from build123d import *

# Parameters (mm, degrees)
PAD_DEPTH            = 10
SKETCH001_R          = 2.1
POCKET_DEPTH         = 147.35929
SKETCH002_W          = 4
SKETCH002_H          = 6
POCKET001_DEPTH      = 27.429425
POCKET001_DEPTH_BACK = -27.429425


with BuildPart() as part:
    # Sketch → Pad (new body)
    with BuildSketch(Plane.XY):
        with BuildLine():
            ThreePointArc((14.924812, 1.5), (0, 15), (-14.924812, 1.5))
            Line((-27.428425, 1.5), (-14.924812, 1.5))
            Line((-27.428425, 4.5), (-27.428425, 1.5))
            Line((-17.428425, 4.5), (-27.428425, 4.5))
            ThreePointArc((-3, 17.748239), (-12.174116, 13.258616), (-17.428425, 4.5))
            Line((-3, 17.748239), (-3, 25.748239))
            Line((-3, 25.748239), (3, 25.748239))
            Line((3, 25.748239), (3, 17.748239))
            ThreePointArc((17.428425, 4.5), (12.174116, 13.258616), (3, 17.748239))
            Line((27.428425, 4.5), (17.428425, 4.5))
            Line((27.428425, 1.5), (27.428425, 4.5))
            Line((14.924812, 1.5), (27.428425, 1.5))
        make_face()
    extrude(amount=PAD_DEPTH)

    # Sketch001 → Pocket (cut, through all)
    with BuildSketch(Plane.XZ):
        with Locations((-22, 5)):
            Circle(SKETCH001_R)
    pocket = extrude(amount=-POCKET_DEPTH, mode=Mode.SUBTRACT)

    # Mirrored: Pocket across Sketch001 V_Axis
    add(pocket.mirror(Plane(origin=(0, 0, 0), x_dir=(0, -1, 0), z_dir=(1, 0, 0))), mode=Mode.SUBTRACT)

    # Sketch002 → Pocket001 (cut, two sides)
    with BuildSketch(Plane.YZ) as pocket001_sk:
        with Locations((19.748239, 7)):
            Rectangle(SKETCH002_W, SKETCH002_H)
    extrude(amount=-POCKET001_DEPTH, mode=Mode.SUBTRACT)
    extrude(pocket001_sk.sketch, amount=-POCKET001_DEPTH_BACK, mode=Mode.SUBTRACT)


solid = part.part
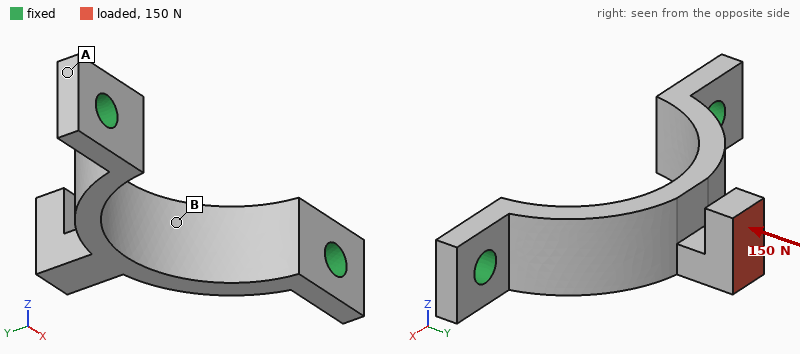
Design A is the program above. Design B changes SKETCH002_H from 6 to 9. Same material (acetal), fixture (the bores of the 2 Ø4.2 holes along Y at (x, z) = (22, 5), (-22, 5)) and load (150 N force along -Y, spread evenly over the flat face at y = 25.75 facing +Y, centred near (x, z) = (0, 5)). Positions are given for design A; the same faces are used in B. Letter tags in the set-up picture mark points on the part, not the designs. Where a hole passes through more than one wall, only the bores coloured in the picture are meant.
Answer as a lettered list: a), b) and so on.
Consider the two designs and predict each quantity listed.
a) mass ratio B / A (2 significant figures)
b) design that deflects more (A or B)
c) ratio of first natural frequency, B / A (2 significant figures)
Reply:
a) 0.98
b) B
c) 0.97
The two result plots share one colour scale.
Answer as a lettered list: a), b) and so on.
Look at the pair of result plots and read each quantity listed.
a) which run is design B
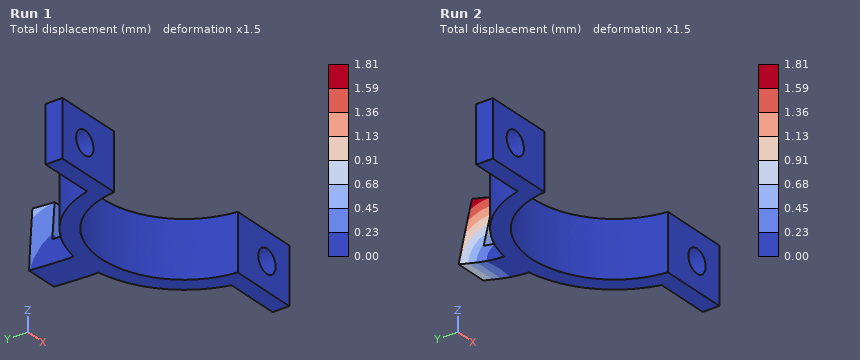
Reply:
a) Run 2
